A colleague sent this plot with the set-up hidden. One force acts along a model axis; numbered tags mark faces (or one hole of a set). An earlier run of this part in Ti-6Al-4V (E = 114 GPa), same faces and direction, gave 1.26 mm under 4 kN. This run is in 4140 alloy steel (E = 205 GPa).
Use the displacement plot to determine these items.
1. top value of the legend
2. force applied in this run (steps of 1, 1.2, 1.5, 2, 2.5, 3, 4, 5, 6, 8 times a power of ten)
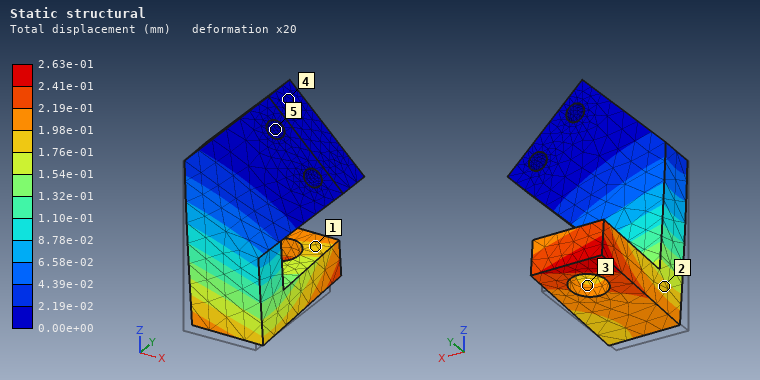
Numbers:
2.63e-01 mm
1.5 kN
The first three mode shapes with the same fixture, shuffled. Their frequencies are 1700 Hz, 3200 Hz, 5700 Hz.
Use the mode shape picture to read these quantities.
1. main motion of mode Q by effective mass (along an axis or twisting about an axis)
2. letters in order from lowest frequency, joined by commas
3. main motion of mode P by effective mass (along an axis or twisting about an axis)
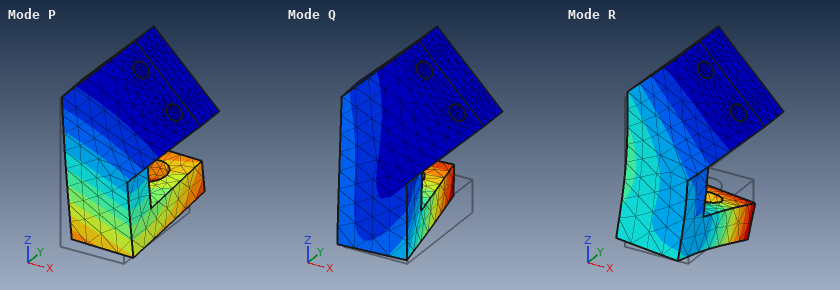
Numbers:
along X
P, Q, R
along Y
